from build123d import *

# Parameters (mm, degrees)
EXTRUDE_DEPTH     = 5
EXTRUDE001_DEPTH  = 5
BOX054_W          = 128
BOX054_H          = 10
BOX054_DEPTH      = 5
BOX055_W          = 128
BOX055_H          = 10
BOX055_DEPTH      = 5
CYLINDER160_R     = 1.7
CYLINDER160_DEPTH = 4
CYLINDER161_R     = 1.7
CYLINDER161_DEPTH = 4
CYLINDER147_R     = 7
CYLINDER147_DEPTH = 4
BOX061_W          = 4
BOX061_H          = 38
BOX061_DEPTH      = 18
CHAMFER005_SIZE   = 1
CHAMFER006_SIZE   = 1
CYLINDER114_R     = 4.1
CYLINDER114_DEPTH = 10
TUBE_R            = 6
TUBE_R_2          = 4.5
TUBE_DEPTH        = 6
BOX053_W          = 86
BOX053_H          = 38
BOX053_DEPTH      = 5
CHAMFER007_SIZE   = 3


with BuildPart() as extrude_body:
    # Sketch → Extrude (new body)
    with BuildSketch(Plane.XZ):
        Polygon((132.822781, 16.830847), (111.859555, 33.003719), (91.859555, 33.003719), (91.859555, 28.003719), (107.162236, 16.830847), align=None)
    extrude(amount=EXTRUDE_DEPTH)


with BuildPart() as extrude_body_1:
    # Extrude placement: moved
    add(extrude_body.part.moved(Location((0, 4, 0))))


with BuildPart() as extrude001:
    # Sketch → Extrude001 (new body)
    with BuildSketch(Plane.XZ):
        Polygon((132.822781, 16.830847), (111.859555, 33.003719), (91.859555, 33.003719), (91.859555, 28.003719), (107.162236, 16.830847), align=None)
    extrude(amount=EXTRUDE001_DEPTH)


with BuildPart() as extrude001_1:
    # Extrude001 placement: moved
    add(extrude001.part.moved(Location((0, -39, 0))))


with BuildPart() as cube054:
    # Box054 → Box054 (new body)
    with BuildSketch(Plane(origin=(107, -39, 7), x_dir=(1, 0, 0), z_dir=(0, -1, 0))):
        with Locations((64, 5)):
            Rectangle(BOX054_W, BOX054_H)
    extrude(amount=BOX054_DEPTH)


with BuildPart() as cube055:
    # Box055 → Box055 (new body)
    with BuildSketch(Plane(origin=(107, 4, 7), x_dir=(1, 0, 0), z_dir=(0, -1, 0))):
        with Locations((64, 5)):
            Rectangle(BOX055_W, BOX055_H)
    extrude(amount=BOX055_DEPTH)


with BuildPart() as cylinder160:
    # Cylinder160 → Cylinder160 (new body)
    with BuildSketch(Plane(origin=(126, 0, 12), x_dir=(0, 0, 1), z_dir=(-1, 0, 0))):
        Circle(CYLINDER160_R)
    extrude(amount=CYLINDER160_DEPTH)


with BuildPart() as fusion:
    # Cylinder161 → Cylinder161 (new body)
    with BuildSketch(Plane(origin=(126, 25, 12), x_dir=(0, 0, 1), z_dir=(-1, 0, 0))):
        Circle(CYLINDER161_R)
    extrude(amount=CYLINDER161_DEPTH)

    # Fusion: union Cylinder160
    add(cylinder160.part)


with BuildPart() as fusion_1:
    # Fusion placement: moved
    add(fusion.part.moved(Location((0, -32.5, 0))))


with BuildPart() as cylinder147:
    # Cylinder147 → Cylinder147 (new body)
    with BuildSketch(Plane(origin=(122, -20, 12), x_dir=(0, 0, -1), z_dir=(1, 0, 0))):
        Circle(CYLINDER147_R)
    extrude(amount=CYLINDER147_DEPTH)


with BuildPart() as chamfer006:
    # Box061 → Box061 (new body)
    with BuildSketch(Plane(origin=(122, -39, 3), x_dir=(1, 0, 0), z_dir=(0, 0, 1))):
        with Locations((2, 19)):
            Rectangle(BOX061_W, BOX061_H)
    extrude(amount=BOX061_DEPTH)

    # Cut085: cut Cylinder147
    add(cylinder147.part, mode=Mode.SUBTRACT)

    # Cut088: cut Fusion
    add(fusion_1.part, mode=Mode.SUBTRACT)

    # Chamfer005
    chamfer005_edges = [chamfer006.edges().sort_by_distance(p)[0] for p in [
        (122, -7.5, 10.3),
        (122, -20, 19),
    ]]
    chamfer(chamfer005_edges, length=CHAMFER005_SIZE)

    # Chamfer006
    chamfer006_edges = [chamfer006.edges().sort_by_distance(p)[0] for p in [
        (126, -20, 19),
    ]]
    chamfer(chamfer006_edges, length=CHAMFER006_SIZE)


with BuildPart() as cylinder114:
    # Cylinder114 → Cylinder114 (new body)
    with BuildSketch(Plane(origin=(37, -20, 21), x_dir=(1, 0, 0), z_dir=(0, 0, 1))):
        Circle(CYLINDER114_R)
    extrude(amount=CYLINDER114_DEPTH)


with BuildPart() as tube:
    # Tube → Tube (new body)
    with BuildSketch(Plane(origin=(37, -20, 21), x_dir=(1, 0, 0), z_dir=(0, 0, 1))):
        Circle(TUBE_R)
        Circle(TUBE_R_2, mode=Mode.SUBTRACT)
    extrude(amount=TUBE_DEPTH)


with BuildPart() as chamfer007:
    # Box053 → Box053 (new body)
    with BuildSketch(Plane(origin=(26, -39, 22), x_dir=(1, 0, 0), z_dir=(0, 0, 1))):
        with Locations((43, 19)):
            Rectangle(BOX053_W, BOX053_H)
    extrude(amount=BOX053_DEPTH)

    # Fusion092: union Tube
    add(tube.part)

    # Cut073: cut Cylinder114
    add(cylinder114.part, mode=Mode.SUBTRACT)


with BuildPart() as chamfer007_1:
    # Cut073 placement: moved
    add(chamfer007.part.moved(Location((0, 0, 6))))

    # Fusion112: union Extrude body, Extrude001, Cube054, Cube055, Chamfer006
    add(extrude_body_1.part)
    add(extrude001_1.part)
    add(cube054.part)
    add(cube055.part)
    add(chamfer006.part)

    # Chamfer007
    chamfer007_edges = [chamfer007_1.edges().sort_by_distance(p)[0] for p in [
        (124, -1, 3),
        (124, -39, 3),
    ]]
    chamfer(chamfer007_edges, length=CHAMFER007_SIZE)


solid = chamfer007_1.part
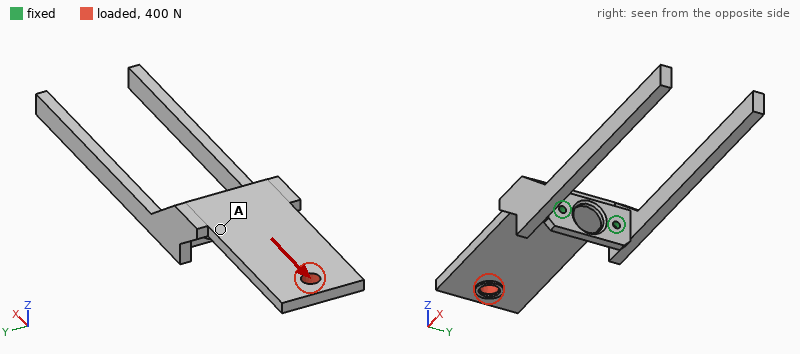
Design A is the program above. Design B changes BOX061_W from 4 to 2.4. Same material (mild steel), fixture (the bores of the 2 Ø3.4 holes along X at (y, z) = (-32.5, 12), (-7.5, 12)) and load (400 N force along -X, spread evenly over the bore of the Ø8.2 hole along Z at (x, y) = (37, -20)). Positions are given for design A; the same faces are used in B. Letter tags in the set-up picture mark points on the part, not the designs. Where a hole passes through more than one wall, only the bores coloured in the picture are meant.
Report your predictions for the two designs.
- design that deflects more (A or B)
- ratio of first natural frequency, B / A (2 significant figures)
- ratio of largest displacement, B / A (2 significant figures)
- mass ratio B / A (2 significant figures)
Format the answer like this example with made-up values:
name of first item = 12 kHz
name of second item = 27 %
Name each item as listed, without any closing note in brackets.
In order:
design that deflects more = B
ratio of first natural frequency, B / A = 0.77
ratio of largest displacement, B / A = 3.4
mass ratio B / A = 0.98
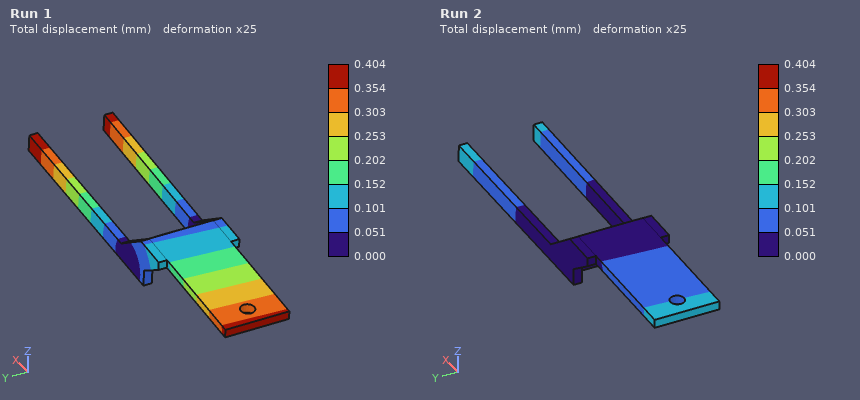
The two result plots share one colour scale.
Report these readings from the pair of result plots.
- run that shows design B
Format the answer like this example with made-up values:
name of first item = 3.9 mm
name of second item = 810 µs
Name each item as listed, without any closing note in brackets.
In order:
run that shows design B = Run 1
